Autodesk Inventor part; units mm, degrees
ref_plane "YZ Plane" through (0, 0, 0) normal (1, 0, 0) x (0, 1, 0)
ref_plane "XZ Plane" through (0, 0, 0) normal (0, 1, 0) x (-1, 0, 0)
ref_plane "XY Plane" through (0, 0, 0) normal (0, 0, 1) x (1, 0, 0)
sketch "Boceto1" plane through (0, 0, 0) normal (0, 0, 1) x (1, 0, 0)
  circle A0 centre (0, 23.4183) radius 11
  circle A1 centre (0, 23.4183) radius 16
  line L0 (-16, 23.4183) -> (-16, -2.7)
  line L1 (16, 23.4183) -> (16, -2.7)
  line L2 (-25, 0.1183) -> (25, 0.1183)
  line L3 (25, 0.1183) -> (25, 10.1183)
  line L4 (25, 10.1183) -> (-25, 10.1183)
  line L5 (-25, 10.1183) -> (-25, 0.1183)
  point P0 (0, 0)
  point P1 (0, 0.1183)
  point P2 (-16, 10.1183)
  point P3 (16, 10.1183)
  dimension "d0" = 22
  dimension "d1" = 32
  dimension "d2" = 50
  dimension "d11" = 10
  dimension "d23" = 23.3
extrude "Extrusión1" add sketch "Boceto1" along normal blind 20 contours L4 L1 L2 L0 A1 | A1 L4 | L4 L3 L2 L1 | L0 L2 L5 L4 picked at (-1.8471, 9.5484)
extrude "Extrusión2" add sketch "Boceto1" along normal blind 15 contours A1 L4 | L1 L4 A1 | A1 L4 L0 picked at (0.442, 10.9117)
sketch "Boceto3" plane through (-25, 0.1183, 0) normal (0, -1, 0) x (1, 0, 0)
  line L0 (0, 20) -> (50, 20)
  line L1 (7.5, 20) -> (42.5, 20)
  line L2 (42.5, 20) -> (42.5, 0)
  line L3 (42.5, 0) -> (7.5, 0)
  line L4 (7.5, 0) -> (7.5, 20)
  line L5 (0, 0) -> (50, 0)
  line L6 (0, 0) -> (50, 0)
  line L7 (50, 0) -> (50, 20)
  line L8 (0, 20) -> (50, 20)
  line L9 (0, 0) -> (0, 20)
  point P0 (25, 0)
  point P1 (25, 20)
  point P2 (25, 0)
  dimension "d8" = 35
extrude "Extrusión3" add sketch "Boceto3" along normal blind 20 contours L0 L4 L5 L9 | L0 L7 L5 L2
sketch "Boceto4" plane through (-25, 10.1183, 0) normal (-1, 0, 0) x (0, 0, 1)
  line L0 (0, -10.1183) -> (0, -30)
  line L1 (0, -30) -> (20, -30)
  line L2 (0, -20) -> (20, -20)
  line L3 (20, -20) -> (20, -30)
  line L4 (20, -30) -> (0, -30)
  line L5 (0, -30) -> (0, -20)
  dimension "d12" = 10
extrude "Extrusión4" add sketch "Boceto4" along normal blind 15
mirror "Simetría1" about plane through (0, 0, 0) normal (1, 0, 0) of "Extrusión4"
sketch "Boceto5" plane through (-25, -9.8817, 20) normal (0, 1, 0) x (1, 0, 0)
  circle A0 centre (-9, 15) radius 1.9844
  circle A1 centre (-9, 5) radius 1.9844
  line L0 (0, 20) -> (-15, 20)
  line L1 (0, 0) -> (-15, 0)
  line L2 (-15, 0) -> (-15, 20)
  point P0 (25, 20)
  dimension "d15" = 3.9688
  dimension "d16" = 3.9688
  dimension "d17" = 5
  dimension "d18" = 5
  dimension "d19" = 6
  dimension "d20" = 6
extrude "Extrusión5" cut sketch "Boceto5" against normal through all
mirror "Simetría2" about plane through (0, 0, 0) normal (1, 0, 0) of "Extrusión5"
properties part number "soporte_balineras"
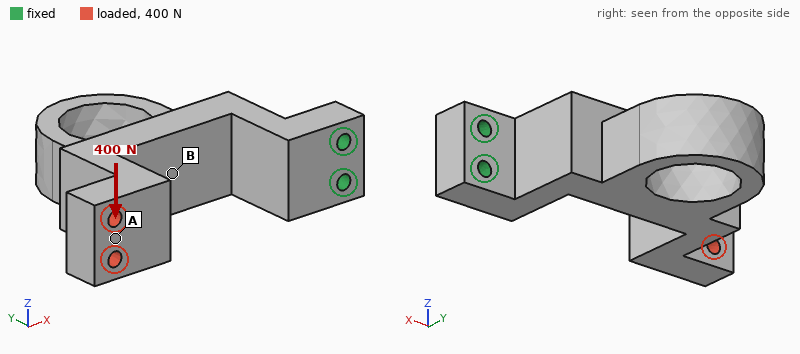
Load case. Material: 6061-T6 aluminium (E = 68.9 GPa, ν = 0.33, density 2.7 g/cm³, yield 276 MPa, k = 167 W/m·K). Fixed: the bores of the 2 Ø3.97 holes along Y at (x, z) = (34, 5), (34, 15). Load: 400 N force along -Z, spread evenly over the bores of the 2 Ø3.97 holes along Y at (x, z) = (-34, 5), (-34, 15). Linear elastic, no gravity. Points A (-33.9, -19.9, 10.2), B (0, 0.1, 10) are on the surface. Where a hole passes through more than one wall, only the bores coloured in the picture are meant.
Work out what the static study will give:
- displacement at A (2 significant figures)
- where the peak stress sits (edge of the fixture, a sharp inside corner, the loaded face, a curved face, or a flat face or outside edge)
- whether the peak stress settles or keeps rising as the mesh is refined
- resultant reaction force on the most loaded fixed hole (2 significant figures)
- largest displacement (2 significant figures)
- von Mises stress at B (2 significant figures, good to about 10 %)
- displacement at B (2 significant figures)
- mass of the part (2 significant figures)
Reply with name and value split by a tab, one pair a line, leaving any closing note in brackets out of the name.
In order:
displacement at A	0.39 mm
where the peak stress sits	a sharp inside corner
whether the peak stress settles or keeps rising as the mesh is refined	keeps rising
resultant reaction force on the most loaded fixed hole	2.2 kN
largest displacement	0.44 mm
von Mises stress at B	22 MPa
displacement at B	0.12 mm
mass of the part	76 g
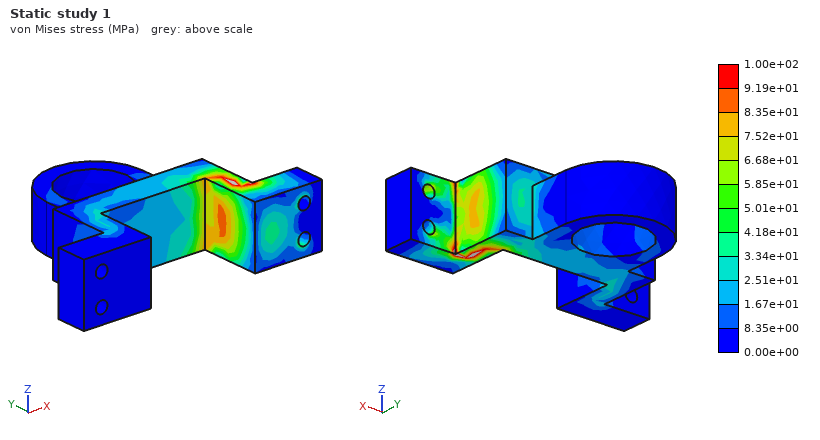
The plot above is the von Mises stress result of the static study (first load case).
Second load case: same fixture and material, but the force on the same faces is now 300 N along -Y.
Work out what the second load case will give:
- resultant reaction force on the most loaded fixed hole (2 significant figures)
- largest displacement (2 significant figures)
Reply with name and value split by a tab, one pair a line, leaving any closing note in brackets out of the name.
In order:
resultant reaction force on the most loaded fixed hole	180 N
largest displacement	0.60 mm
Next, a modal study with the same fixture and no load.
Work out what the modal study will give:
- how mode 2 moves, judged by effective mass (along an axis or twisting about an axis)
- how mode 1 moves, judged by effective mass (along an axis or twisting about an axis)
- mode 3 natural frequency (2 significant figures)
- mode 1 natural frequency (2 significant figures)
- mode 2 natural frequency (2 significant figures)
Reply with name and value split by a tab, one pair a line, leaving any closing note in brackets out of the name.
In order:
how mode 2 moves, judged by effective mass	along Z
how mode 1 moves, judged by effective mass	along Y
mode 3 natural frequency	2400 Hz
mode 1 natural frequency	750 Hz
mode 2 natural frequency	1200 Hz
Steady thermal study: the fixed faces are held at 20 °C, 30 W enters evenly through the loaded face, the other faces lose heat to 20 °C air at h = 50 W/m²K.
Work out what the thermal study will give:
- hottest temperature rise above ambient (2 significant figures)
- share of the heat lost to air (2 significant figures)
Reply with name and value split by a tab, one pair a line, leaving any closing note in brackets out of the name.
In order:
hottest temperature rise above ambient	62 K
share of the heat lost to air	43 %
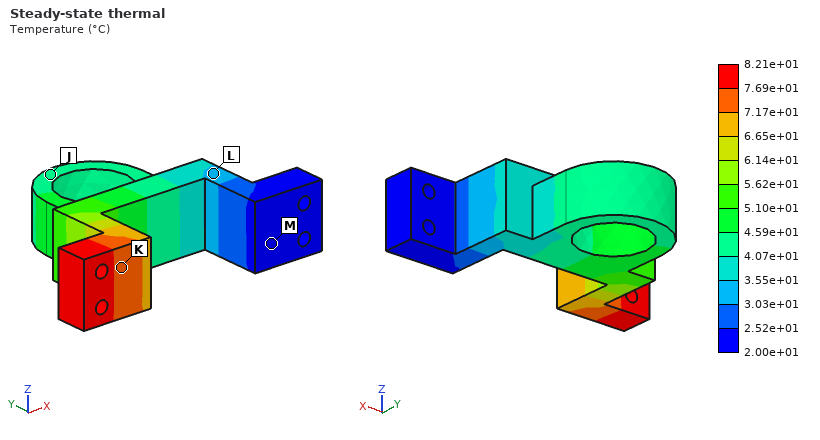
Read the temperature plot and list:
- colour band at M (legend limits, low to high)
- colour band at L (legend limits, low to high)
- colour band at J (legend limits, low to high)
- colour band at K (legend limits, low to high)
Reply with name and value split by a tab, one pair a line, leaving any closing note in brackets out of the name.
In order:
colour band at M	2.00e+01 to 2.52e+01 °C
colour band at L	3.03e+01 to 3.55e+01 °C
colour band at J	4.07e+01 to 4.59e+01 °C
colour band at K	7.17e+01 to 7.69e+01 °C
